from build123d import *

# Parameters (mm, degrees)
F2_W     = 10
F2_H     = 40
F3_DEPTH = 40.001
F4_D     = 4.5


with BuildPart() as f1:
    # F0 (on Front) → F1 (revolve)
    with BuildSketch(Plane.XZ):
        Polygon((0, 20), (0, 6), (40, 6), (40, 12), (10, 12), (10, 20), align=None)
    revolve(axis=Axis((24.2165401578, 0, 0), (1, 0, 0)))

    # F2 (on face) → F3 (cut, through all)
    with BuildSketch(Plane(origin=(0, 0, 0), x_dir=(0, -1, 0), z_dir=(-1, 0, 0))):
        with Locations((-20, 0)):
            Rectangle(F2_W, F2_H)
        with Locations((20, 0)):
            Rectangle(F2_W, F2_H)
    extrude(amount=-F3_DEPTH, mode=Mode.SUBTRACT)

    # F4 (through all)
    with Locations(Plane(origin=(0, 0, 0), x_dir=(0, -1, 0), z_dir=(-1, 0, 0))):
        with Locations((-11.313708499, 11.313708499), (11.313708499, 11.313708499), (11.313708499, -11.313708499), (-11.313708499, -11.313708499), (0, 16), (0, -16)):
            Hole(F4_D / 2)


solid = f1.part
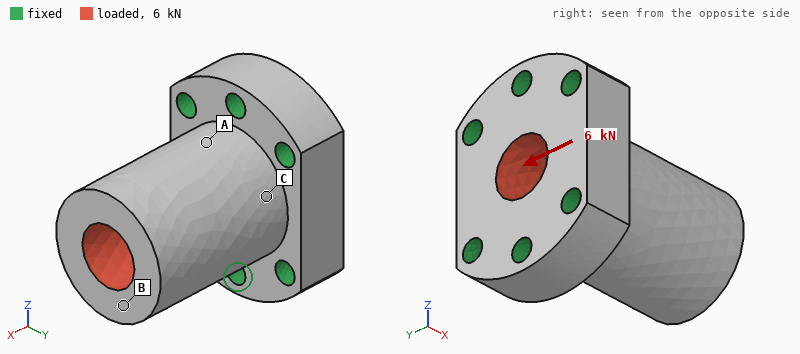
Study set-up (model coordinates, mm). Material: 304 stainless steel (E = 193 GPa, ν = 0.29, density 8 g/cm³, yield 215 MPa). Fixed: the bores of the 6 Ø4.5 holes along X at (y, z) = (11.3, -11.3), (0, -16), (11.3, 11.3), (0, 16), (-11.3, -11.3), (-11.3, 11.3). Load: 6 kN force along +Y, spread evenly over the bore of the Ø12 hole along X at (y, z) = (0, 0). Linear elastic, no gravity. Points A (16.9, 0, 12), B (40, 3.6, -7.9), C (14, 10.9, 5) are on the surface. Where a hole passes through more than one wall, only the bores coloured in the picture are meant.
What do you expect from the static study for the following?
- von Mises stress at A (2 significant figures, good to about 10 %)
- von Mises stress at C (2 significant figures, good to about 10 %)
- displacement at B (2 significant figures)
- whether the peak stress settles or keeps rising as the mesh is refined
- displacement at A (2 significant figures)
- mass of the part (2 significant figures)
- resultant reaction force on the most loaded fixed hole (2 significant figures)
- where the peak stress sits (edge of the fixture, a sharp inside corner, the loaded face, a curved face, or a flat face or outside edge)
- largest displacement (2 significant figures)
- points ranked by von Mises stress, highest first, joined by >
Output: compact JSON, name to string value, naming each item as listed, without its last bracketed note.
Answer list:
{"von Mises stress at A": "22 MPa", "von Mises stress at C": "39 MPa", "displacement at B": "16 µm", "whether the peak stress settles or keeps rising as the mesh is refined": "keeps rising", "displacement at A": "4.1 µm", "mass of the part": "150 g", "resultant reaction force on the most loaded fixed hole": "2.4 kN", "where the peak stress sits": "edge of the fixture", "largest displacement": "17 µm", "points ranked by von Mises stress, highest first, joined by >": "C > A > B"}
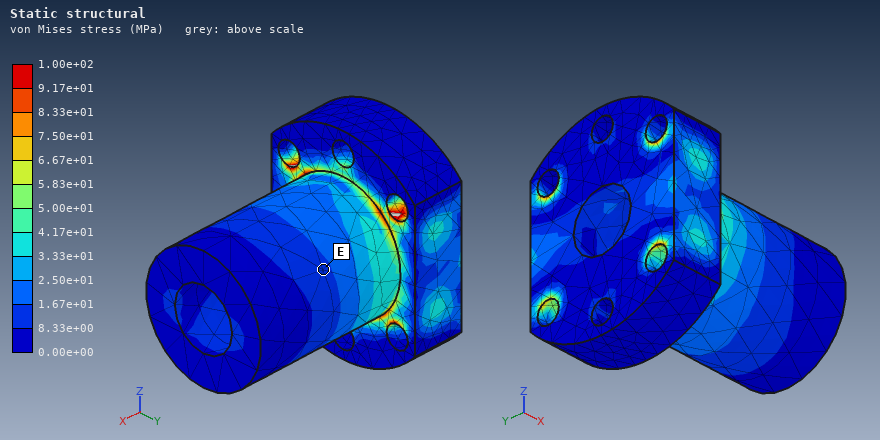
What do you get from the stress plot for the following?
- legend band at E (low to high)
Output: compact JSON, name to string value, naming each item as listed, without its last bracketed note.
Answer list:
{"legend band at E": "8.33e+00 to 1.67e+01 MPa"}
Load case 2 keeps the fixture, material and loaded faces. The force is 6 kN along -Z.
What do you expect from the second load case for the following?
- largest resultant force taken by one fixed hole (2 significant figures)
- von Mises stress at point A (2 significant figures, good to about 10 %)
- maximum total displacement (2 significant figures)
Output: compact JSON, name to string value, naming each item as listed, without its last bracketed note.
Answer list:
{"largest resultant force taken by one fixed hole": "2.0 kN", "von Mises stress at point A": "29 MPa", "maximum total displacement": "14 µm"}
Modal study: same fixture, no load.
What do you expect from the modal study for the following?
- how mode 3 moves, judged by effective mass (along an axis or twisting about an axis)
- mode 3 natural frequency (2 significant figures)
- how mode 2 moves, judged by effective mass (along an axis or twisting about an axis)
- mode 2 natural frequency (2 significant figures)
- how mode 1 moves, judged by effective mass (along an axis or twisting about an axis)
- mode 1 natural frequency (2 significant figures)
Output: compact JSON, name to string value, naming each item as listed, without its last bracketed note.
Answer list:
{"how mode 3 moves, judged by effective mass": "twisting about X", "mode 3 natural frequency": "23 kHz", "how mode 2 moves, judged by effective mass": "along Z", "mode 2 natural frequency": "12 kHz", "how mode 1 moves, judged by effective mass": "along Y", "mode 1 natural frequency": "11 kHz"}
